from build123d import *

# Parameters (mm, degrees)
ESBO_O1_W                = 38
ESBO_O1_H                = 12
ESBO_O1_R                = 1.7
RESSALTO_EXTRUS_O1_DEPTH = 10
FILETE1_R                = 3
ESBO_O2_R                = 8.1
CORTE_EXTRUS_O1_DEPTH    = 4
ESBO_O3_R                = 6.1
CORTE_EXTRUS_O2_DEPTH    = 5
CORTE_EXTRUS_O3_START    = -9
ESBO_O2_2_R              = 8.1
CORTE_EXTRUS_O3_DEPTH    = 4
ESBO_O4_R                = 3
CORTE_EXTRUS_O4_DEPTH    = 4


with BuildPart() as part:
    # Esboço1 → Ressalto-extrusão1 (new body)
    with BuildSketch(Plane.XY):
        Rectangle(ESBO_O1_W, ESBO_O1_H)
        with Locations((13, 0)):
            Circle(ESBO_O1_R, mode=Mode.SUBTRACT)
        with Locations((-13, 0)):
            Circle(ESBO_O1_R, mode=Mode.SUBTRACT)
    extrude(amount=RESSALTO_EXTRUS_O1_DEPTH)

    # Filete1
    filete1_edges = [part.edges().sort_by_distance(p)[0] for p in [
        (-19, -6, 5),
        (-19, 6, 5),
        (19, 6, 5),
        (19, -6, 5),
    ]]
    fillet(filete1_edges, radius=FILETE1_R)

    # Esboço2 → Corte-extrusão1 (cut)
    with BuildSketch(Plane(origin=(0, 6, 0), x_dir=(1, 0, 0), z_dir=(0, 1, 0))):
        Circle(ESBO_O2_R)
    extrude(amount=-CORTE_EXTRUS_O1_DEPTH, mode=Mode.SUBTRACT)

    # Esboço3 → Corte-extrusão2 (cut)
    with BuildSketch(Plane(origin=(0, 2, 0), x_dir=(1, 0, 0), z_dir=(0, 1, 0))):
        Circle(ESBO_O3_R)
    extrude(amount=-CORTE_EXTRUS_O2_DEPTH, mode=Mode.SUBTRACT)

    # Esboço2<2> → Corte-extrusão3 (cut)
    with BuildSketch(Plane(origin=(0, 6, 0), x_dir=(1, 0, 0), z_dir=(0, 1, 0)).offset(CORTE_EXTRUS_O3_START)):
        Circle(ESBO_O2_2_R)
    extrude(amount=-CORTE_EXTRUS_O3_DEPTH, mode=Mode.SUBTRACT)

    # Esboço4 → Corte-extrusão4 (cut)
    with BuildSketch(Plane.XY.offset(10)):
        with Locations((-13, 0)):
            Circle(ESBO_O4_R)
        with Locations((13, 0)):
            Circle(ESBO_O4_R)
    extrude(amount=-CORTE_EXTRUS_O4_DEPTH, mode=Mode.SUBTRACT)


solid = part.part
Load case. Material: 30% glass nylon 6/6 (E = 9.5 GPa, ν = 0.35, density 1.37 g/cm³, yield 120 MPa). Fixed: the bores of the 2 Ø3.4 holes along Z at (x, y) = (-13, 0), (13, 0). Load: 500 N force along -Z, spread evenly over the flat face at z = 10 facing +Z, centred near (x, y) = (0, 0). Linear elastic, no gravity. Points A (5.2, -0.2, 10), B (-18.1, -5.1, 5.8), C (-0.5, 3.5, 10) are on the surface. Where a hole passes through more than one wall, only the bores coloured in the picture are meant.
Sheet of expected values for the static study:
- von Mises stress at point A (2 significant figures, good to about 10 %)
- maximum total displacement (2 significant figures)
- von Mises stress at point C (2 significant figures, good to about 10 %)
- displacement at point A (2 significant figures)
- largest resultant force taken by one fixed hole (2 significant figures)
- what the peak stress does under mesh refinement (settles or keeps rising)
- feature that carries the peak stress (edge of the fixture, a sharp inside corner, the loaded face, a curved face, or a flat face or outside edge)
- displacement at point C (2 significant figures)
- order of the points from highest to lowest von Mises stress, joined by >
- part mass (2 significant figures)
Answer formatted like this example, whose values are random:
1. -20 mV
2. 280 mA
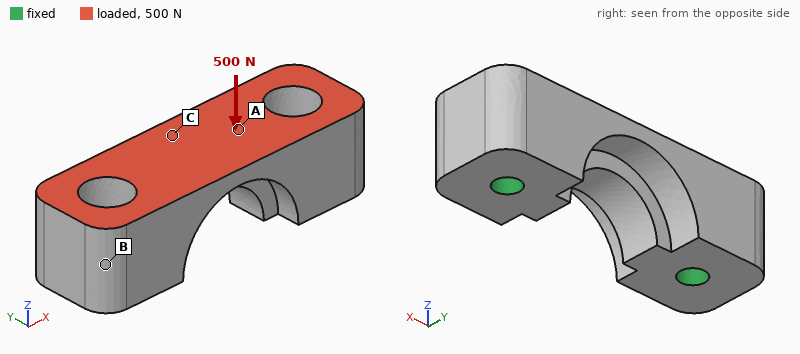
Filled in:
1. 2.6 MPa
2. 14 µm
3. 6.9 MPa
4. 7.9 µm
5. 270 N
6. keeps rising
7. edge of the fixture
8. 12 µm
9. C > A > B
10. 4.3 g
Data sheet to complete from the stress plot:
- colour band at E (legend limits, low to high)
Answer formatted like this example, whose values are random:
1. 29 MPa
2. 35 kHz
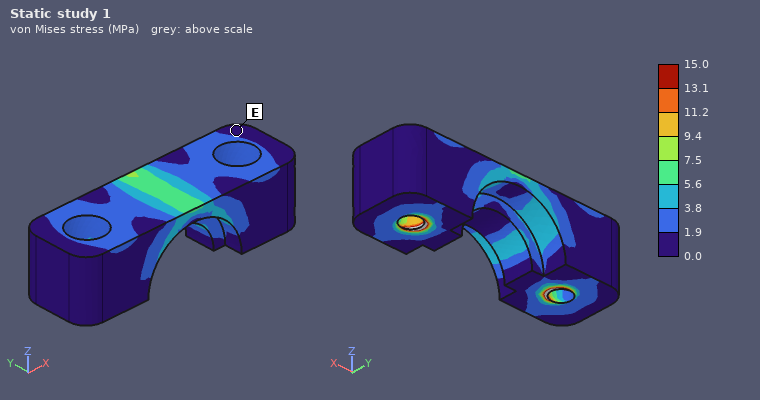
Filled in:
1. 0.0 to 1.9 MPa
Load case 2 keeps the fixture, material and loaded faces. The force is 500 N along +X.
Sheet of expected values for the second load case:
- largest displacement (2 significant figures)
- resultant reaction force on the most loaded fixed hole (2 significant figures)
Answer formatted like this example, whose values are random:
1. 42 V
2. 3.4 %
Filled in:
1. 12 µm
2. 260 N
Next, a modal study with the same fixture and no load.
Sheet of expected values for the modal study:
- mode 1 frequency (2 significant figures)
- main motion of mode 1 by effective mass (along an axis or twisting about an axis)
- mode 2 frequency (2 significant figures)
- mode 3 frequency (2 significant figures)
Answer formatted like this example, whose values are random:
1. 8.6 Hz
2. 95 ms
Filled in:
1. 17 kHz
2. along Y
3. 25 kHz
4. 25 kHz
